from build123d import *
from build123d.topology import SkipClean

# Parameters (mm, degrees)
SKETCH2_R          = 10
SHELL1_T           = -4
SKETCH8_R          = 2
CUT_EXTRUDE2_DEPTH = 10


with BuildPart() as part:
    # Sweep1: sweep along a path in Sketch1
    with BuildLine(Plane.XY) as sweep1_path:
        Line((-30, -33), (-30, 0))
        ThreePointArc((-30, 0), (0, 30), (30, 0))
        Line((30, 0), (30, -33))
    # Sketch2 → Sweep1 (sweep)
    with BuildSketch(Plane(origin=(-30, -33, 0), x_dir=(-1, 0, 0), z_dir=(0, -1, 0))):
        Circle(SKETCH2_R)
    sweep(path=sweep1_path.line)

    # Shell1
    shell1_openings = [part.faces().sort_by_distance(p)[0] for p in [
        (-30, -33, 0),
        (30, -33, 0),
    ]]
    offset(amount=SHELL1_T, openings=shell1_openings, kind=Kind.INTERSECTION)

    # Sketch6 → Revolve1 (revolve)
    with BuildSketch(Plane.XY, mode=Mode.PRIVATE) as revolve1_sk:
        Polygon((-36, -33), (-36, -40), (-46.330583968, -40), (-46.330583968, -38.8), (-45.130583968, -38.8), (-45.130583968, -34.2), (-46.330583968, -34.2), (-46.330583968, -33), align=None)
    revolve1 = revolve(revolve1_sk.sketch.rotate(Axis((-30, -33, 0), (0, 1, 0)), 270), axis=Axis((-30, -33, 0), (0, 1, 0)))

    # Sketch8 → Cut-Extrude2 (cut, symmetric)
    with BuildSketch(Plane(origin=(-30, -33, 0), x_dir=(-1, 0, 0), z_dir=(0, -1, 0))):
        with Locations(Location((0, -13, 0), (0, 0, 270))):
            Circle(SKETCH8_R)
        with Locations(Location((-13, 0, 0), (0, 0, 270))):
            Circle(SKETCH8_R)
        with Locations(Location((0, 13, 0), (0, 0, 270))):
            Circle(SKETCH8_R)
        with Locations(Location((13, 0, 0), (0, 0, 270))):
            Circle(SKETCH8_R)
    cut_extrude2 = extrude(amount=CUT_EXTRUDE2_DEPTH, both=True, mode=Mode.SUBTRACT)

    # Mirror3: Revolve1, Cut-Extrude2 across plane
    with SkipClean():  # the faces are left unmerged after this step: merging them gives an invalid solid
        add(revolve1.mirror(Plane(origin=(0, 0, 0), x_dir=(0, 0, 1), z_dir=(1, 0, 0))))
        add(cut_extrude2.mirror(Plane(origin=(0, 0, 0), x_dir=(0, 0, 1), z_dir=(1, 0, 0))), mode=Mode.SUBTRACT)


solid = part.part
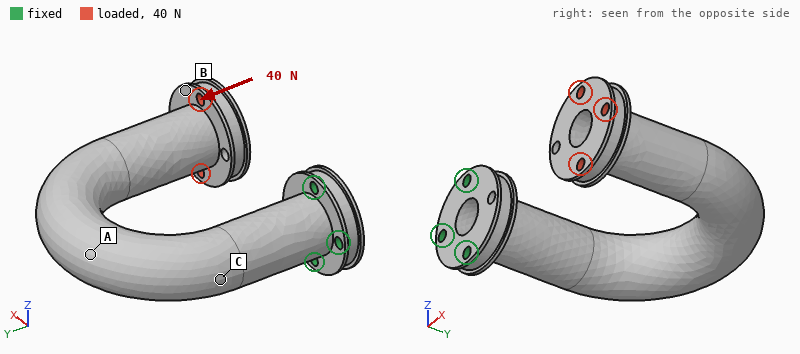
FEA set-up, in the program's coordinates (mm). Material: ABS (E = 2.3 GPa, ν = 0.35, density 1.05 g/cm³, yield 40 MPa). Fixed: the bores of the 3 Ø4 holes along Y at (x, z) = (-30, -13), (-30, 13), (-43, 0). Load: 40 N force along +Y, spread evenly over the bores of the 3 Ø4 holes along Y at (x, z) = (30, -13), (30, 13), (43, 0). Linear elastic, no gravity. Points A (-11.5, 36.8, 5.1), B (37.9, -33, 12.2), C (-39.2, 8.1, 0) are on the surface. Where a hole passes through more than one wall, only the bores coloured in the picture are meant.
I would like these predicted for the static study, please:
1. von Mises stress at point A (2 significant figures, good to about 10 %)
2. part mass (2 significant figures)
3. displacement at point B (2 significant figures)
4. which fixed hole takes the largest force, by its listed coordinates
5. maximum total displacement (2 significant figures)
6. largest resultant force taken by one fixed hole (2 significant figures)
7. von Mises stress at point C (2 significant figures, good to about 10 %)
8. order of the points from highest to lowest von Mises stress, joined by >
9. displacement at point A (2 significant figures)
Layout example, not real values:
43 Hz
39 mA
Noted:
2.1 MPa
43 g
1.2 mm
(-43, 0)
1.4 mm
140 N
3.1 MPa
C > A > B
0.68 mm
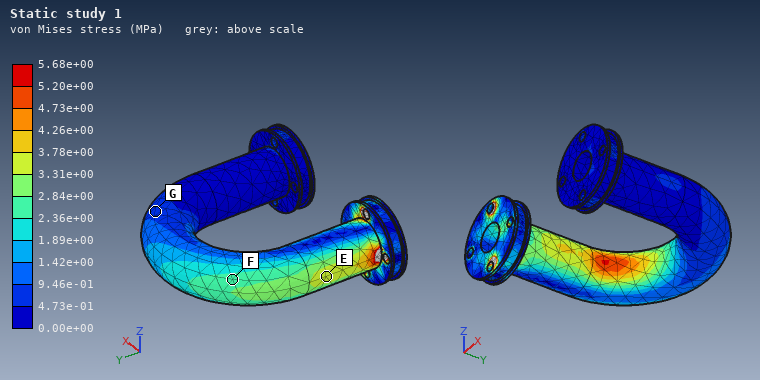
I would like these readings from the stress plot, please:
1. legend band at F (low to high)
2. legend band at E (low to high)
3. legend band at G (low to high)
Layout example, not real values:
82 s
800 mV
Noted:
2.36e+00 to 2.84e+00 MPa
3.31e+00 to 3.78e+00 MPa
4.73e-01 to 9.46e-01 MPa
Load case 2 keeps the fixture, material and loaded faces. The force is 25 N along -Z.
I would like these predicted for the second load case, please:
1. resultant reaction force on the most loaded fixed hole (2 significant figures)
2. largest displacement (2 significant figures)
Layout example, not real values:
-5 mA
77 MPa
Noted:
55 N
1.5 mm
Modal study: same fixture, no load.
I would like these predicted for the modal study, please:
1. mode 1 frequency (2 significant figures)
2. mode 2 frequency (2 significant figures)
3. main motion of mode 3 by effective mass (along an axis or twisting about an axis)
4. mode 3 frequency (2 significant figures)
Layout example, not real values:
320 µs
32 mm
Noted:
210 Hz
210 Hz
along X
370 Hz
